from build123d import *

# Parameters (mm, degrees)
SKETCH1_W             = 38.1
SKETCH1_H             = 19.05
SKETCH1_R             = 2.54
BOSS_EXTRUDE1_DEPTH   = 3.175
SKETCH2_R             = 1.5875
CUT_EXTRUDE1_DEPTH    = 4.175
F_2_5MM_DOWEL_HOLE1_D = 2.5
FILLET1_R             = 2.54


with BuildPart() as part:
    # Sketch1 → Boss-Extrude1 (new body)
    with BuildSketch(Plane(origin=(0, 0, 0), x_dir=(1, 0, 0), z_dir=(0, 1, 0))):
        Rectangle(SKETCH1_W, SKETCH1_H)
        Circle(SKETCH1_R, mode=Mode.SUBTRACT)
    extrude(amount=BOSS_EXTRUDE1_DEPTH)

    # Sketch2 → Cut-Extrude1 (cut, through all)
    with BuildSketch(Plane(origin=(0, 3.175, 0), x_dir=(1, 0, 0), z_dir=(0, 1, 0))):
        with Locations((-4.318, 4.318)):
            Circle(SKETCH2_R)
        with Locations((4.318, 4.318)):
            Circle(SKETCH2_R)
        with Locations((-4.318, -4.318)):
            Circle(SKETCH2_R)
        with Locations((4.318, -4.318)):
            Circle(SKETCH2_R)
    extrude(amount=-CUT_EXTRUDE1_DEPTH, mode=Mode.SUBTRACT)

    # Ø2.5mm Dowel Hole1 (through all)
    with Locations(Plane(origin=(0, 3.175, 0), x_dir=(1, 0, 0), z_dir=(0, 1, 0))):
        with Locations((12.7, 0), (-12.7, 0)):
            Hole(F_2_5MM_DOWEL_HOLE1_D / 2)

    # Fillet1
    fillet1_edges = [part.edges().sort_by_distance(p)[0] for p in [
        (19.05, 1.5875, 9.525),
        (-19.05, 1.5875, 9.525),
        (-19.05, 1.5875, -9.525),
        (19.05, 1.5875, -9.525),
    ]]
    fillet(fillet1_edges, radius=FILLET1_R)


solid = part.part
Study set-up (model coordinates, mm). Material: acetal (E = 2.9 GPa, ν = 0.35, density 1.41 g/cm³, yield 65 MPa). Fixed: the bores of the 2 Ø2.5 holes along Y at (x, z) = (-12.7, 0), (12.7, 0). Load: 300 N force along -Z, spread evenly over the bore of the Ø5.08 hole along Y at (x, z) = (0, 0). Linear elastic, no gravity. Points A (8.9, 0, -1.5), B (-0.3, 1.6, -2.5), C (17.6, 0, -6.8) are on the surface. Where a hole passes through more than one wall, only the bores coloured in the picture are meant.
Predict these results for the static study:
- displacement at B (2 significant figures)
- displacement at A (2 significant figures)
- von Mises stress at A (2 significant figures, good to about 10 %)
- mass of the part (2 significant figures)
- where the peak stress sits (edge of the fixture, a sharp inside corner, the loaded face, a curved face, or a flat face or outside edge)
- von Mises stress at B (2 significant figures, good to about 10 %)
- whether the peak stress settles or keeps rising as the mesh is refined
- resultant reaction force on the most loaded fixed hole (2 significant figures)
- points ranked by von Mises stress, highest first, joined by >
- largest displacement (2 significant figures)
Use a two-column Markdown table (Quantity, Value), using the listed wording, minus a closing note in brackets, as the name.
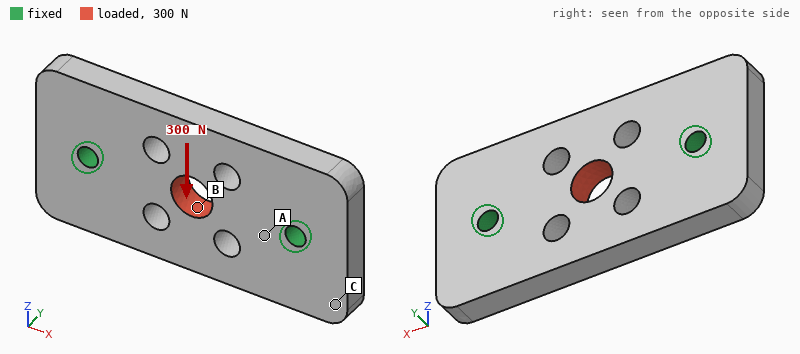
| Quantity | Value |
|---|---|
| displacement at B | 61 µm |
| displacement at A | 19 µm |
| von Mises stress at A | 4.9 MPa |
| mass of the part | 2.9 g |
| where the peak stress sits | edge of the fixture |
| von Mises stress at B | 9.3 MPa |
| whether the peak stress settles or keeps rising as the mesh is refined | keeps rising |
| resultant reaction force on the most loaded fixed hole | 150 N |
| points ranked by von Mises stress, highest first, joined by > | B > A > C |
| largest displacement | 62 µm |
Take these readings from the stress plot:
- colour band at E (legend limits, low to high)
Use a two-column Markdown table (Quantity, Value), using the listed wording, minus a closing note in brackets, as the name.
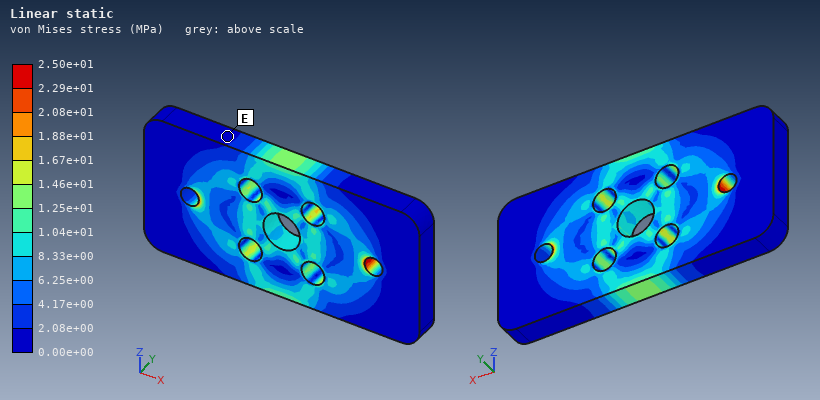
| Quantity | Value |
|---|---|
| colour band at E | 0.00e+00 to 2.08e+00 MPa |
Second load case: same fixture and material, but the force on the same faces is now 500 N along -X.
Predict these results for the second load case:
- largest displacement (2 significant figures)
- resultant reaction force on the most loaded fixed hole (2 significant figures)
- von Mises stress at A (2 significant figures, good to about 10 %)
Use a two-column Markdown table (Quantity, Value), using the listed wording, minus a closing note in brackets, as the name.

| Quantity | Value |
|---|---|
| largest displacement | 47 µm |
| resultant reaction force on the most loaded fixed hole | 250 N |
| von Mises stress at A | 11 MPa |
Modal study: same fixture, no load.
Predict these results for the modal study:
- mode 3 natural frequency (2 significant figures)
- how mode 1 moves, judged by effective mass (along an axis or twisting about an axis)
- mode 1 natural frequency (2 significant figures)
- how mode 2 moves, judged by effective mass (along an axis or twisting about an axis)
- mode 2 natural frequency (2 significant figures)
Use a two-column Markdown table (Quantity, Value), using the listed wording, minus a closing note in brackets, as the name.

| Quantity | Value |
|---|---|
| mode 3 natural frequency | 7300 Hz |
| how mode 1 moves, judged by effective mass | twisting about X |
| mode 1 natural frequency | 4800 Hz |
| how mode 2 moves, judged by effective mass | along Y |
| mode 2 natural frequency | 5200 Hz |
